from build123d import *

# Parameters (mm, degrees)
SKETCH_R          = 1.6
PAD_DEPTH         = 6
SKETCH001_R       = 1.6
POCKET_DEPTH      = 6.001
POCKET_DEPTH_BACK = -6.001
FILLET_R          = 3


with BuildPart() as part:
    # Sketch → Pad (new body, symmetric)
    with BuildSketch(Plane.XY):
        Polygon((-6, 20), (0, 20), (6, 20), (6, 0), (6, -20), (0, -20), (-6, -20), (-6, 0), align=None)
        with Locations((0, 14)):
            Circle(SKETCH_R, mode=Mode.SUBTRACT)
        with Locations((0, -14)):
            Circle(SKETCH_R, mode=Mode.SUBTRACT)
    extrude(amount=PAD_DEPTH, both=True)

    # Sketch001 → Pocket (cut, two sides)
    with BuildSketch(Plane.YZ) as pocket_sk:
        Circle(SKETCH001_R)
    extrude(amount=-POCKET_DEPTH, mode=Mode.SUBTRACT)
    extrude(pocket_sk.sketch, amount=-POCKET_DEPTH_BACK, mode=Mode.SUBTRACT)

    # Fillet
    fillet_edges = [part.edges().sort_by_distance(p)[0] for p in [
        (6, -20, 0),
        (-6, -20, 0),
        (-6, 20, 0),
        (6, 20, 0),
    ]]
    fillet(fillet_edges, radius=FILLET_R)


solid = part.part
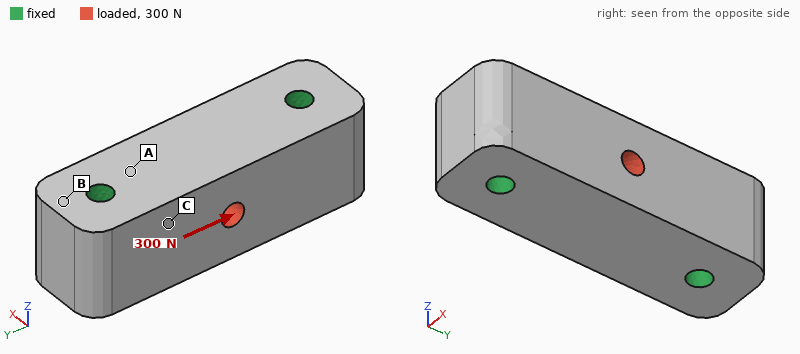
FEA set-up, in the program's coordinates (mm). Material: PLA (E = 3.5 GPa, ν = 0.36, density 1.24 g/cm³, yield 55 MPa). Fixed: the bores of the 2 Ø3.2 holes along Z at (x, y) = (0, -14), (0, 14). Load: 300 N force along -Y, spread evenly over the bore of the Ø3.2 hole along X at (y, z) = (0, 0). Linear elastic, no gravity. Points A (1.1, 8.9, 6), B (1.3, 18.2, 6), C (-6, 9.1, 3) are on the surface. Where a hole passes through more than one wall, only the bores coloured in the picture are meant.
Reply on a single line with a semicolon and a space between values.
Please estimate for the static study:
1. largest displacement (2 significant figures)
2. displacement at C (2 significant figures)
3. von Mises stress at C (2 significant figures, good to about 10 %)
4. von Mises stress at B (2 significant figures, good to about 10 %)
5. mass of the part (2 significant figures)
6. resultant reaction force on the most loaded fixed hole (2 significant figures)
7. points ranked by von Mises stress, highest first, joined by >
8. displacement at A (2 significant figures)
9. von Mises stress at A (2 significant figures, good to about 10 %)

5.8 µm; 2.3 µm; 0.76 MPa; 0.40 MPa; 6.7 g; 150 N; A > C > B; 1.9 µm; 1.2 MPa
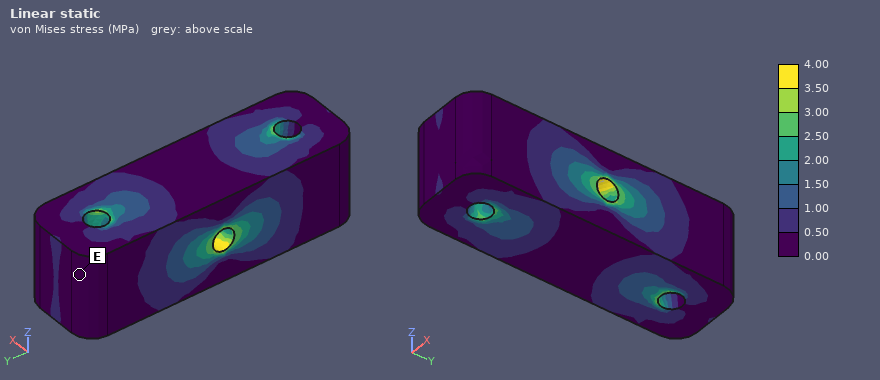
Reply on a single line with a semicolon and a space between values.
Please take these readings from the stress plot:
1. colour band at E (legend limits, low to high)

0.00 to 0.50 MPa
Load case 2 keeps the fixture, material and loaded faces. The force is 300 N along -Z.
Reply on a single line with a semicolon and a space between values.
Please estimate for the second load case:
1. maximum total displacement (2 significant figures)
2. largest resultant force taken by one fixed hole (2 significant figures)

20 µm; 150 N
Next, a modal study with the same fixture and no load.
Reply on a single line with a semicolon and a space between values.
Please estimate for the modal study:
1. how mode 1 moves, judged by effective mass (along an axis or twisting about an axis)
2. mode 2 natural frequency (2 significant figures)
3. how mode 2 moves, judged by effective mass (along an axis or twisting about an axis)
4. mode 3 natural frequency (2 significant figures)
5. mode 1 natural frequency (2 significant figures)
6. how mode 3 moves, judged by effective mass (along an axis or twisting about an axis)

along X; 14 kHz; along Z; 17 kHz; 12 kHz; twisting about Y
